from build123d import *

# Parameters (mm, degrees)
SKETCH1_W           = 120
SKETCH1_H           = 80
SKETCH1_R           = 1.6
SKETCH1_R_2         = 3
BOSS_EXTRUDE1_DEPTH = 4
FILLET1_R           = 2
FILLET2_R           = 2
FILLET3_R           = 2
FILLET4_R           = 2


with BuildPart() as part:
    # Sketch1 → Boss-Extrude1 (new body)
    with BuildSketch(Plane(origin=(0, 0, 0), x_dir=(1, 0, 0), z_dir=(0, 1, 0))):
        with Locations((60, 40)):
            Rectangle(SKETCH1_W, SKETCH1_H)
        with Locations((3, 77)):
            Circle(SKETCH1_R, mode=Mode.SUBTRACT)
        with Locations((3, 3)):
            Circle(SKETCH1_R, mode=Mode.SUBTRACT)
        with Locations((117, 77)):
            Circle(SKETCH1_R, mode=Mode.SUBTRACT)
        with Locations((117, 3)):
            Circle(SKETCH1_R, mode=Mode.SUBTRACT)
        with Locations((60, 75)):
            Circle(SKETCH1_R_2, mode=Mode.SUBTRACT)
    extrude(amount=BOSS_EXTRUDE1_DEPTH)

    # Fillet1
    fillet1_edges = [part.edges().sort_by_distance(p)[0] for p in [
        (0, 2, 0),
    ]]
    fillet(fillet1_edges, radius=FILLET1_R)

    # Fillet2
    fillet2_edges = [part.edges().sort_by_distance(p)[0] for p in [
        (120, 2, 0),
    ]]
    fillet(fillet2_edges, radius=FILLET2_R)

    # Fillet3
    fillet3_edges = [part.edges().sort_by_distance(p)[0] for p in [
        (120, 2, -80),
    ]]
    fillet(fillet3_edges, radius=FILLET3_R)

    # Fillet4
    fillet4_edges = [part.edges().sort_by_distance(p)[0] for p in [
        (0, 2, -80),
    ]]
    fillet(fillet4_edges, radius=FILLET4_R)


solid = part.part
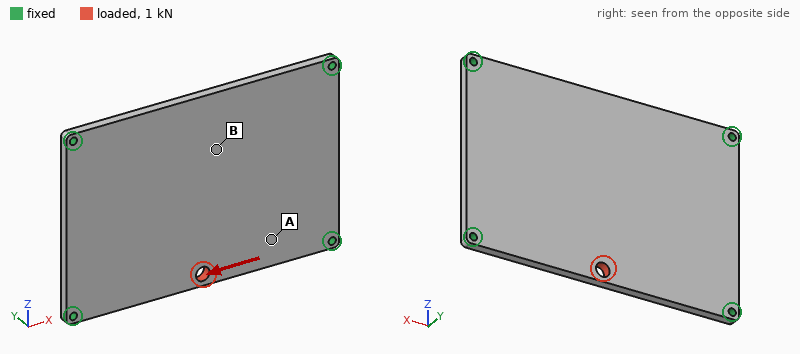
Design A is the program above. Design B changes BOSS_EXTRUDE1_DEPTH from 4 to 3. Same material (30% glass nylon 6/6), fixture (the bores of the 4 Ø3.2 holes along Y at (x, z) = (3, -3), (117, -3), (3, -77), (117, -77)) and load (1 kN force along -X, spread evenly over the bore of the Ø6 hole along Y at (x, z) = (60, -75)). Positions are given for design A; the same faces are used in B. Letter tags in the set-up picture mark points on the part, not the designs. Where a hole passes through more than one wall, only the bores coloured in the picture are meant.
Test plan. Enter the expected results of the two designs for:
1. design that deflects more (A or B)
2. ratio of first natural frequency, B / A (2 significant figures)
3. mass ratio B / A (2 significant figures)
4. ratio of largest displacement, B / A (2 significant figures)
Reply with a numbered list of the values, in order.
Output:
1. B
2. 0.77
3. 0.75
4. 1.3
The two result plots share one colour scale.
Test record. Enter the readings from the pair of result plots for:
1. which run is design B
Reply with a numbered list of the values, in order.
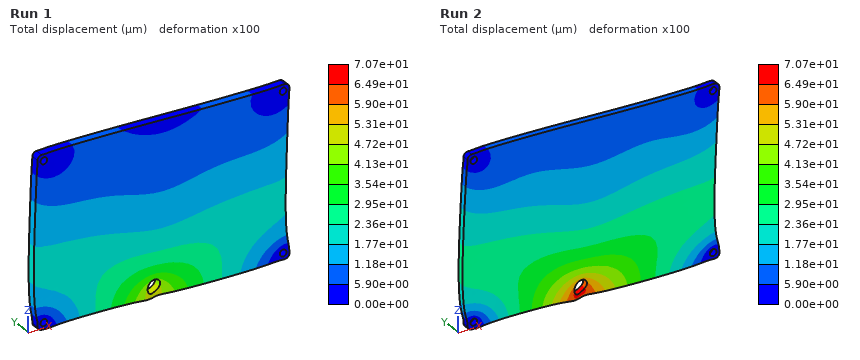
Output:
1. Run 2
